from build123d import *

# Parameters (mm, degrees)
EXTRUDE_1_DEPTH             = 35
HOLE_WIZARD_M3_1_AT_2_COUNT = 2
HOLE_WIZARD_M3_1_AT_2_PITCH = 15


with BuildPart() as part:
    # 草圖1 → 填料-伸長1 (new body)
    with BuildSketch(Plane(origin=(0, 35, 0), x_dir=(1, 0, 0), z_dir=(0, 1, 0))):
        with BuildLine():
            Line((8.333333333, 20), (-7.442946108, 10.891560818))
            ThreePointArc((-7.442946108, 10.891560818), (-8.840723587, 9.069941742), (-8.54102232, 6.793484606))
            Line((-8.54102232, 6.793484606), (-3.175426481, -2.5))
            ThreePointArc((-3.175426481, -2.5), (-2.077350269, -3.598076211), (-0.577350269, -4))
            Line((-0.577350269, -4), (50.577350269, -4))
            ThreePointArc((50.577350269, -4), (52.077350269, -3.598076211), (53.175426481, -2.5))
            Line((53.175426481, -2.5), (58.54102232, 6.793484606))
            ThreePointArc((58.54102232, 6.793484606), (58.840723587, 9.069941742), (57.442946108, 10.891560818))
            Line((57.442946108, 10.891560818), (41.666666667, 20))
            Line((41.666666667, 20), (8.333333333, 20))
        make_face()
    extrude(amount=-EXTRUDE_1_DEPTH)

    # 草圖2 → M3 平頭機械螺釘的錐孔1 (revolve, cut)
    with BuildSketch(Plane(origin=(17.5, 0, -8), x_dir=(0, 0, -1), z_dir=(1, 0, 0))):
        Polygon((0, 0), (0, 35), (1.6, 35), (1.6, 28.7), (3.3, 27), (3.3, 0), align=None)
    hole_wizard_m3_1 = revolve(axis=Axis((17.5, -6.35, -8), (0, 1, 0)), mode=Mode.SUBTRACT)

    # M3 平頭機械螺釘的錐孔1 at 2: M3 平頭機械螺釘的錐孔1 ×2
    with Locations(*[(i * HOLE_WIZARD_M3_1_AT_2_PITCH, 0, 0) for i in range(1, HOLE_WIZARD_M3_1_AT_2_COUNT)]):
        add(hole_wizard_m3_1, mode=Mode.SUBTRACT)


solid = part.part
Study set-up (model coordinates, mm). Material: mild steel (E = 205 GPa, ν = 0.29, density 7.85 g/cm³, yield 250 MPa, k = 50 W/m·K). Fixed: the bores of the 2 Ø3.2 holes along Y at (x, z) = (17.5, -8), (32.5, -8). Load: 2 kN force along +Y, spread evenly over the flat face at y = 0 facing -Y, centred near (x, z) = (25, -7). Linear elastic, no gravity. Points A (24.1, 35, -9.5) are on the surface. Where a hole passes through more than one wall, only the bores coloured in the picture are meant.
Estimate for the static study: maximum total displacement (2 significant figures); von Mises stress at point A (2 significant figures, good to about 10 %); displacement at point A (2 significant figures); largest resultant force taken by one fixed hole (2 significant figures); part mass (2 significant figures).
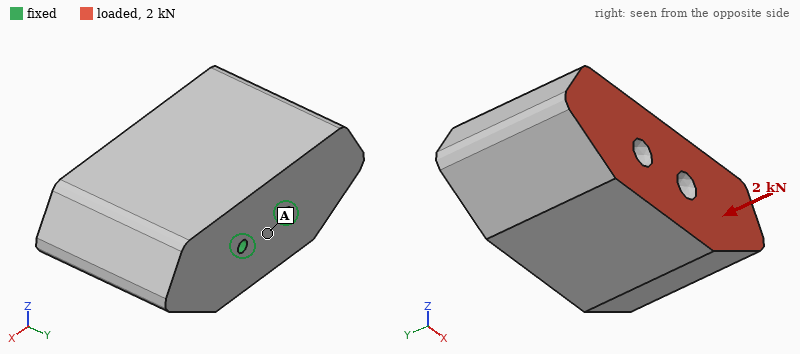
1.5 µm
4.9 MPa
0.31 µm
1.0 kN
360 g
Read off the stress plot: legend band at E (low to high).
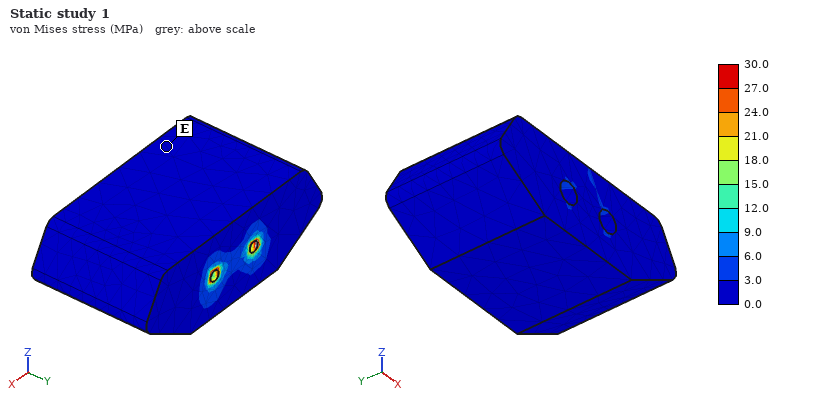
0.0 to 3.0 MPa
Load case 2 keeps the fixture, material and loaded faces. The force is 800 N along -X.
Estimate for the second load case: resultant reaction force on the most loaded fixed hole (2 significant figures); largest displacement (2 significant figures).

1.4 kN
5.5 µm
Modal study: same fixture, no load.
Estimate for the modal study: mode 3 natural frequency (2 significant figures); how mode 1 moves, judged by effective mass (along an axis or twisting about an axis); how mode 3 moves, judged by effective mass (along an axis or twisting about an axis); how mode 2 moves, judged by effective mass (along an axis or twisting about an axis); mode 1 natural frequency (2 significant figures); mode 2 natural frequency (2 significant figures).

6900 Hz
along Z
twisting about Y
along X
3200 Hz
5100 Hz
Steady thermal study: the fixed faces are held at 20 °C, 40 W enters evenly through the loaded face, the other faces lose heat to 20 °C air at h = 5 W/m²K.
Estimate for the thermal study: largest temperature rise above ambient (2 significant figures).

34 K
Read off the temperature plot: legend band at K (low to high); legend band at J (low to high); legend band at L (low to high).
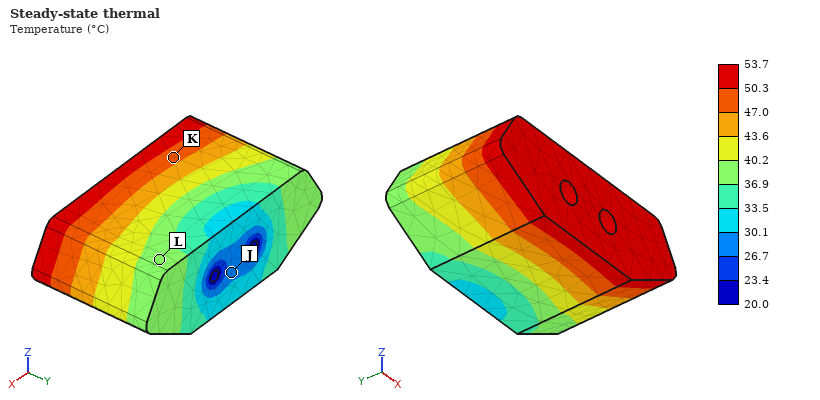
47.0 to 50.3 °C
26.7 to 30.1 °C
36.9 to 40.2 °C
